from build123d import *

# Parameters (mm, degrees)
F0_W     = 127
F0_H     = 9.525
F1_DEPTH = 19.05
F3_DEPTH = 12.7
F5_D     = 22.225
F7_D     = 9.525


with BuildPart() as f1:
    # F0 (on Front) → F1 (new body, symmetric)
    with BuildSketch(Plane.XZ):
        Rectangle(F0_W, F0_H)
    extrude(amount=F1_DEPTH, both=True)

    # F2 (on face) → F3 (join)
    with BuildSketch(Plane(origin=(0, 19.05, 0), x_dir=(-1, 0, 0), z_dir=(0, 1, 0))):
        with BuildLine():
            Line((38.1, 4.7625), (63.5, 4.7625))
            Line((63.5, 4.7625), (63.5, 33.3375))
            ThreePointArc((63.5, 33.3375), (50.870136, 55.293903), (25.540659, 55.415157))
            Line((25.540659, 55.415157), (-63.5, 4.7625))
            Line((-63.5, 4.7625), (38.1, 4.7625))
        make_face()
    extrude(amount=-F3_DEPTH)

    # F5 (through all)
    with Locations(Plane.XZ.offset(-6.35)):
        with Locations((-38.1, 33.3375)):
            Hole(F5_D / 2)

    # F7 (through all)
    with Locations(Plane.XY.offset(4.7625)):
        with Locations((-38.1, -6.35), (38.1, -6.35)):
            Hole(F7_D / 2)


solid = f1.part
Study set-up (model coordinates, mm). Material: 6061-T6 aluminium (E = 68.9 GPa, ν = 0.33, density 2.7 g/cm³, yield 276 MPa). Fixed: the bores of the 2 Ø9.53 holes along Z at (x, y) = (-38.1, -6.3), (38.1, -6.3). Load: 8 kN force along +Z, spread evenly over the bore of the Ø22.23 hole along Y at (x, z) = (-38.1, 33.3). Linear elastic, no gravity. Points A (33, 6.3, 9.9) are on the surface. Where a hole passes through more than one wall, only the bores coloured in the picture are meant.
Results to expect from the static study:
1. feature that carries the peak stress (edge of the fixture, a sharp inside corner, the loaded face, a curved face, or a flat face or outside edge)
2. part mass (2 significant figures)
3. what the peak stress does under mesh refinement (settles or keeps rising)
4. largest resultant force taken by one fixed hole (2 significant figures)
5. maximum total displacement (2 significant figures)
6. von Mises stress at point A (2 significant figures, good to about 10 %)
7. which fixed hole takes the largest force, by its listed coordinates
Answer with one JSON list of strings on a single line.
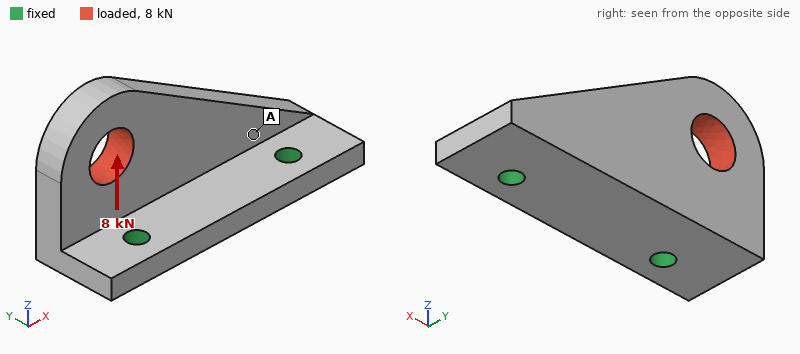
["edge of the fixture", "250 g", "keeps rising", "7.7 kN", "0.26 mm", "17 MPa", "(-38.1, -6.3)"]
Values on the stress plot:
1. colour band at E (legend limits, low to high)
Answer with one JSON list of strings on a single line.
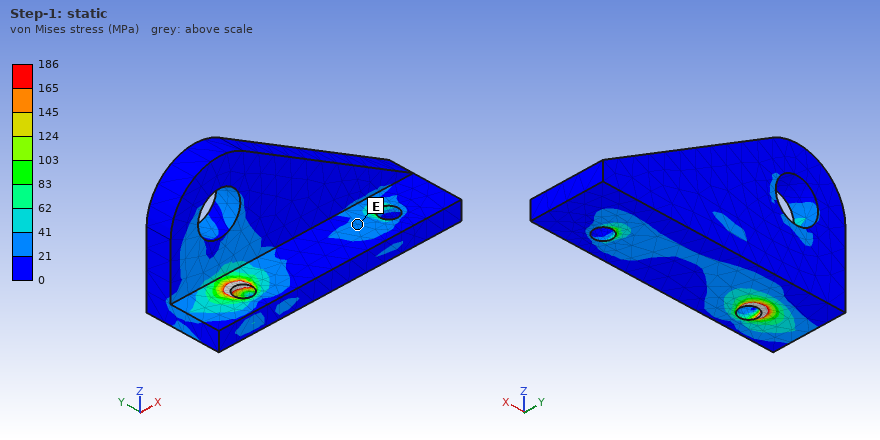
["21 to 41 MPa"]
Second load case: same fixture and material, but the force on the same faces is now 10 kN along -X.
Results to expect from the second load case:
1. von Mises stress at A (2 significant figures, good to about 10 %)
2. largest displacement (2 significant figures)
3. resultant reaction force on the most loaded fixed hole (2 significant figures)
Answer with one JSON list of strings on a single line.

["44 MPa", "0.11 mm", "6.9 kN"]
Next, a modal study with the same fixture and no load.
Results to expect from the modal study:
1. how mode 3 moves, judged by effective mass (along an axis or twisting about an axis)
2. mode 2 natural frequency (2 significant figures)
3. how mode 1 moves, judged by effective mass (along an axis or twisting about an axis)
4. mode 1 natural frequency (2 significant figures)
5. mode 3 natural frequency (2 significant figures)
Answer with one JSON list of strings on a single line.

["along Z", "4900 Hz", "along Y", "2100 Hz", "6200 Hz"]
